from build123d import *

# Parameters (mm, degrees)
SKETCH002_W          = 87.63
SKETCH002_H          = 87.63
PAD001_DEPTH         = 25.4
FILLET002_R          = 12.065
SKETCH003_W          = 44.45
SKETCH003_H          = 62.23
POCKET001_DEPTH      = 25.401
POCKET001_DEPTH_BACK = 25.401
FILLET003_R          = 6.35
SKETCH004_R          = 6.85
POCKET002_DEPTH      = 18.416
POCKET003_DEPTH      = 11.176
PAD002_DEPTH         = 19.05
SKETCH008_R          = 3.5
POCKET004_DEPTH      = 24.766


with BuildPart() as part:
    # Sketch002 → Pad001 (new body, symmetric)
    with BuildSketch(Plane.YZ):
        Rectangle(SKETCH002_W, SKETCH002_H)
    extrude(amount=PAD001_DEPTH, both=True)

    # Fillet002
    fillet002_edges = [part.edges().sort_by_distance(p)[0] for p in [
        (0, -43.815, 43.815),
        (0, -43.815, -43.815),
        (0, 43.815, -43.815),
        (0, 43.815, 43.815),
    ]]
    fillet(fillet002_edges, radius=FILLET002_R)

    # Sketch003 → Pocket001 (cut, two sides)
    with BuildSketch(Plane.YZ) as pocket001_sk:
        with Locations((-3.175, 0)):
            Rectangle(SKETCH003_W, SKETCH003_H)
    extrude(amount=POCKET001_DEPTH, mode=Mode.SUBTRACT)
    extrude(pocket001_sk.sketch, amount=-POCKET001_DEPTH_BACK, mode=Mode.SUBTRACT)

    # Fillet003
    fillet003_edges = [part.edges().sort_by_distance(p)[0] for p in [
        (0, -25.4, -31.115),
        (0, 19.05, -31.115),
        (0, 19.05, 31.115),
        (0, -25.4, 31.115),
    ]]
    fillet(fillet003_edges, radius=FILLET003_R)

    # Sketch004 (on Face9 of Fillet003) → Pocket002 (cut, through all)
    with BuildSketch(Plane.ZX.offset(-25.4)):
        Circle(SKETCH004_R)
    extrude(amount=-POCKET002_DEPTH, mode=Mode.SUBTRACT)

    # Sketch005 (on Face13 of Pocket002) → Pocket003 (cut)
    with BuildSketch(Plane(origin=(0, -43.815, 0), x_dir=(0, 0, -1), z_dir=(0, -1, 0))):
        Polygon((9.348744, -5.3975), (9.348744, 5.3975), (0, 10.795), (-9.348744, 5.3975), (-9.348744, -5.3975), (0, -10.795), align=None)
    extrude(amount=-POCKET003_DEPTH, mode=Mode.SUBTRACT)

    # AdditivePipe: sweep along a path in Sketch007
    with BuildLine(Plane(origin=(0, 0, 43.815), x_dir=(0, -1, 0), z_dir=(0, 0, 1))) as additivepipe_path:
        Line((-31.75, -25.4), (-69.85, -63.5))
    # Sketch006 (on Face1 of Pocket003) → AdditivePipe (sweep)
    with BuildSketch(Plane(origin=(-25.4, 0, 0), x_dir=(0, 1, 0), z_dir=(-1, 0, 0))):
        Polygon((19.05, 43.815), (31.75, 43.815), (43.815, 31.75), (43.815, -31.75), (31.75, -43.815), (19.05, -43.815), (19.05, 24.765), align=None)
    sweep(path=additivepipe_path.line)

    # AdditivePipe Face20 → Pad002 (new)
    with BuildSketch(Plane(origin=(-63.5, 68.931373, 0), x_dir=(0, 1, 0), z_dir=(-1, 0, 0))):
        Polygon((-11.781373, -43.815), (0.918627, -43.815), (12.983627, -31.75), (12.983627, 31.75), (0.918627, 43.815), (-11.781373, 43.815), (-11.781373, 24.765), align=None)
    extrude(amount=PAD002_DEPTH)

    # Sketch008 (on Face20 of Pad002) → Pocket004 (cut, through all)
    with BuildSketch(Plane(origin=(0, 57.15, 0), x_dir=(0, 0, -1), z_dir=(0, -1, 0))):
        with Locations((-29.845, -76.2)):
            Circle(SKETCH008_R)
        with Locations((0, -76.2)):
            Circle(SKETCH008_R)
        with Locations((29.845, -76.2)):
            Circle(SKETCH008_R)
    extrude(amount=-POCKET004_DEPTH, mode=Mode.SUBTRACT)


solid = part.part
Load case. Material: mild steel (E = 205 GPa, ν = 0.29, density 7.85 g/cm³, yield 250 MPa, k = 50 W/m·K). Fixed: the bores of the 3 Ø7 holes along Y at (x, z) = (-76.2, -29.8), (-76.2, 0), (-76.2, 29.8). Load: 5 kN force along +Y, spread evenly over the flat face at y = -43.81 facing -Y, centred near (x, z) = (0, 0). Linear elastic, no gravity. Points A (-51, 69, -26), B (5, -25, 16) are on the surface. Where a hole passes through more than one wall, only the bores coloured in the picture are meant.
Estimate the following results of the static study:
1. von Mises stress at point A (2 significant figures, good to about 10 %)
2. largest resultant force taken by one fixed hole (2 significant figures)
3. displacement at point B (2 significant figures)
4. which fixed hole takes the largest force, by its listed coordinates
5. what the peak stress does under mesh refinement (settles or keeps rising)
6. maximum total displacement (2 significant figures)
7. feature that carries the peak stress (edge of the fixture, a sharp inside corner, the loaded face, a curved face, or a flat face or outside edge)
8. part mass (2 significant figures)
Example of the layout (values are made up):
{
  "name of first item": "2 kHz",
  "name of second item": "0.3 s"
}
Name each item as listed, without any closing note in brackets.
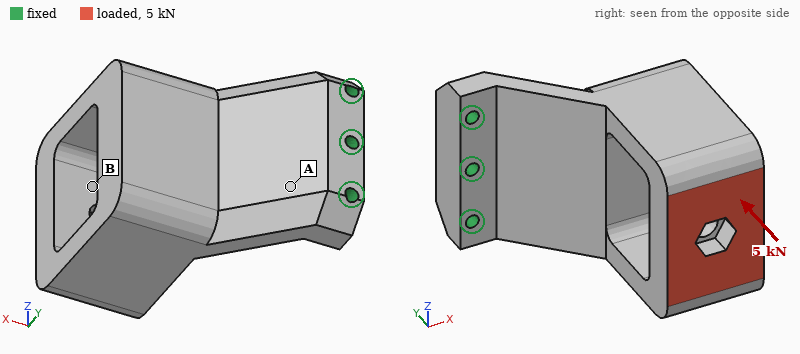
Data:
{
  "von Mises stress at point A": "67 MPa",
  "largest resultant force taken by one fixed hole": "2.8 kN",
  "displacement at point B": "0.18 mm",
  "which fixed hole takes the largest force, by its listed coordinates": "(-76.2, 0)",
  "what the peak stress does under mesh refinement": "keeps rising",
  "maximum total displacement": "0.23 mm",
  "feature that carries the peak stress": "edge of the fixture",
  "part mass": "2.8 kg"
}
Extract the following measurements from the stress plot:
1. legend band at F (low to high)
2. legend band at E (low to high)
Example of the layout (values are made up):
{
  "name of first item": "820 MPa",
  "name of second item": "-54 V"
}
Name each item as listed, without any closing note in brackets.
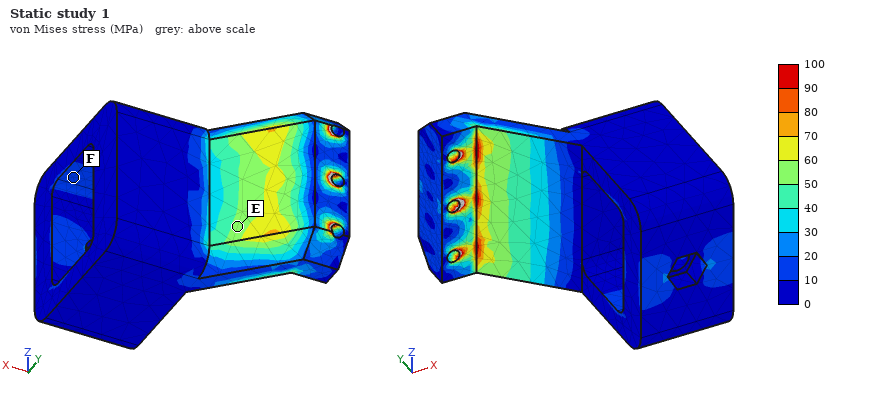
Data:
{
  "legend band at F": "10 to 20 MPa",
  "legend band at E": "50 to 60 MPa"
}
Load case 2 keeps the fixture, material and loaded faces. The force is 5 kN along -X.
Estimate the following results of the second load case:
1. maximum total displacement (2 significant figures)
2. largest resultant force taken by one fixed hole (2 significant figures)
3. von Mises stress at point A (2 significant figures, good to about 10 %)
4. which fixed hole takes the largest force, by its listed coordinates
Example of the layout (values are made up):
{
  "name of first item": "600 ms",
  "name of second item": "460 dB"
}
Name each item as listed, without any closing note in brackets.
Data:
{
  "maximum total displacement": "0.48 mm",
  "largest resultant force taken by one fixed hole": "3.2 kN",
  "von Mises stress at point A": "120 MPa",
  "which fixed hole takes the largest force, by its listed coordinates": "(-76.2, 0)"
}
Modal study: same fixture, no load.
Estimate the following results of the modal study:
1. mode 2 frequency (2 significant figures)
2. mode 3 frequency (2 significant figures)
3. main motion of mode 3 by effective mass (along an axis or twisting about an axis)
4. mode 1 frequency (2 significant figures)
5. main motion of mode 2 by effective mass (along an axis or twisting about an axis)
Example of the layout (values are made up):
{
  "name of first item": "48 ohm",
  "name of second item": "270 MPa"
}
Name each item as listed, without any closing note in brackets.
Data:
{
  "mode 2 frequency": "1300 Hz",
  "mode 3 frequency": "2100 Hz",
  "main motion of mode 3 by effective mass": "along Z",
  "mode 1 frequency": "530 Hz",
  "main motion of mode 2 by effective mass": "along Z"
}
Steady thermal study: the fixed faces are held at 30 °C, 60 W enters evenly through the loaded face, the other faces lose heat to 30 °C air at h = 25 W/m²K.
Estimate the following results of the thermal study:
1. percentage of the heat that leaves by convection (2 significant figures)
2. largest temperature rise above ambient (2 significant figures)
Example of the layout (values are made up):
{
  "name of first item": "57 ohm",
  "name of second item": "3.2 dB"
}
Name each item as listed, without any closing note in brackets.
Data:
{
  "percentage of the heat that leaves by convection": "61 %",
  "largest temperature rise above ambient": "70 K"
}
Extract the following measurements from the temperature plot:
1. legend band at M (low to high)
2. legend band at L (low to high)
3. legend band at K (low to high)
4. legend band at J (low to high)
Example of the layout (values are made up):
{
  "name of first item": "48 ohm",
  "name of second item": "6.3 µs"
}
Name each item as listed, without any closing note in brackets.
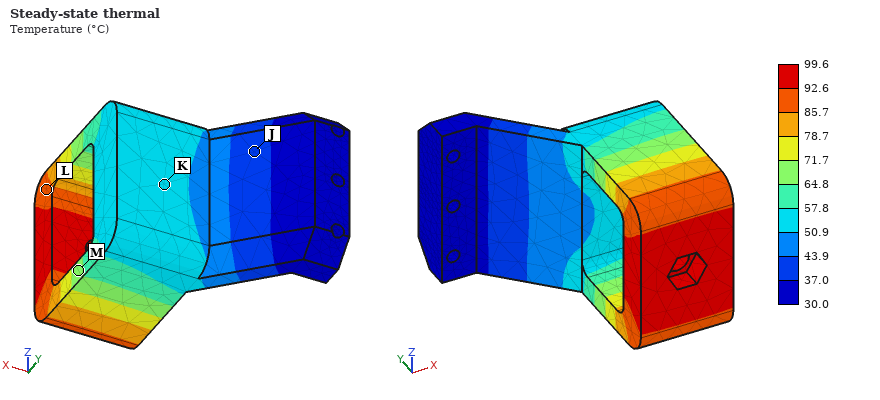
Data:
{
  "legend band at M": "64.8 to 71.7 °C",
  "legend band at L": "85.7 to 92.6 °C",
  "legend band at K": "50.9 to 57.8 °C",
  "legend band at J": "37.0 to 43.9 °C"
}
